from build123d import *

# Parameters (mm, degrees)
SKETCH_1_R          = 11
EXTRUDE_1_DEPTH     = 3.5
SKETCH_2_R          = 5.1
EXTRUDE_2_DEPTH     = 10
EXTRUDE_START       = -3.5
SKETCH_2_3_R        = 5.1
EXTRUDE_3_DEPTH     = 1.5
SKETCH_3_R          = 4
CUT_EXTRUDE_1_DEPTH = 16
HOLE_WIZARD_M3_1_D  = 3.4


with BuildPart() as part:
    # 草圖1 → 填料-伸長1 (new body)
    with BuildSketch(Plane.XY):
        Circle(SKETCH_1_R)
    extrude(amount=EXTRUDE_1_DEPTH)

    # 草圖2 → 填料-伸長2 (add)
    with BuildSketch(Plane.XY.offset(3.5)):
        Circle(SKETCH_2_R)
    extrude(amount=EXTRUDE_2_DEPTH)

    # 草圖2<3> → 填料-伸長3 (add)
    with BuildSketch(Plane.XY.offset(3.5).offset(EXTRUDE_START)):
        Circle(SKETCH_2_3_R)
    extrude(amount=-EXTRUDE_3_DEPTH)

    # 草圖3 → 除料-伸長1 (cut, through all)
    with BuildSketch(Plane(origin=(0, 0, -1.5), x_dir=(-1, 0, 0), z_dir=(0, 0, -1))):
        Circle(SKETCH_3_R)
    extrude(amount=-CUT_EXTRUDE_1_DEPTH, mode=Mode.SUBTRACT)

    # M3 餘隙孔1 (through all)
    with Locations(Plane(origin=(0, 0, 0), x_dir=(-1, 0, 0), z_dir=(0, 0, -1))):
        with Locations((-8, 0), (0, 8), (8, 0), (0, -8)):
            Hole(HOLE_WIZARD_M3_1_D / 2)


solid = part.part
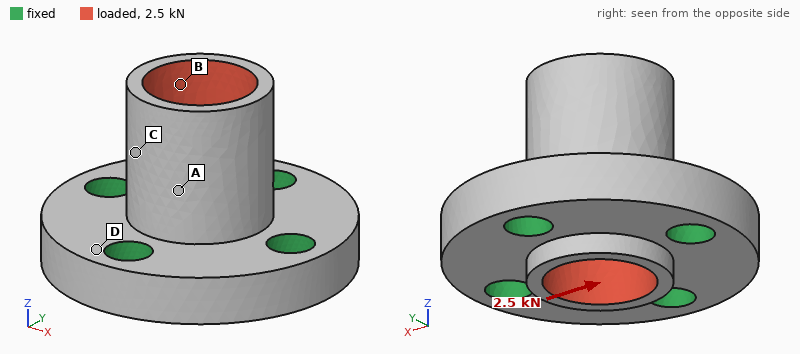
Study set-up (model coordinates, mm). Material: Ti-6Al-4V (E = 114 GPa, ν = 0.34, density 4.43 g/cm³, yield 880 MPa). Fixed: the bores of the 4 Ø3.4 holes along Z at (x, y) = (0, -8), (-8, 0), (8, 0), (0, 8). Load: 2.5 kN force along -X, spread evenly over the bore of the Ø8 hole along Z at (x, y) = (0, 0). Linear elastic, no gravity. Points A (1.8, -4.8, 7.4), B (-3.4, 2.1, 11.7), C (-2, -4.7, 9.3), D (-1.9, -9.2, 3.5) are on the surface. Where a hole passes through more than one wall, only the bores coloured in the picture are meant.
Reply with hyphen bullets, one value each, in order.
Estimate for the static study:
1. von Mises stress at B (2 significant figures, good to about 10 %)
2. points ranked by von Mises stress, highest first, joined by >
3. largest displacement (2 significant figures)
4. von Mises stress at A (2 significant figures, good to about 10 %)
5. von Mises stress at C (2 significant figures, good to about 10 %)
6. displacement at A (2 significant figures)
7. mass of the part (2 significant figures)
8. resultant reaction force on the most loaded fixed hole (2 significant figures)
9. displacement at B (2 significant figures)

- 35 MPa
- A > C > B > D
- 26 µm
- 92 MPa
- 69 MPa
- 12 µm
- 6.2 g
- 1.0 kN
- 23 µm
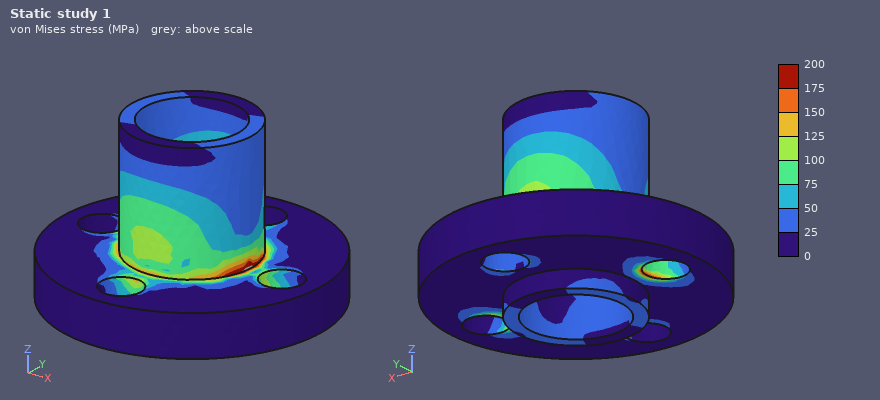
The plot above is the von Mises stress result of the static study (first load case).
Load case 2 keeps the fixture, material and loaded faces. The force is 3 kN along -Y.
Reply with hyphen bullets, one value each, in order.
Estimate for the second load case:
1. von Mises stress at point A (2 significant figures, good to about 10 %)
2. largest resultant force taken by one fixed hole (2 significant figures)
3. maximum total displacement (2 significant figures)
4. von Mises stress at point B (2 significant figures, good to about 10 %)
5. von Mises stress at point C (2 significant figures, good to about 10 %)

- 61 MPa
- 1.3 kN
- 32 µm
- 45 MPa
- 51 MPa
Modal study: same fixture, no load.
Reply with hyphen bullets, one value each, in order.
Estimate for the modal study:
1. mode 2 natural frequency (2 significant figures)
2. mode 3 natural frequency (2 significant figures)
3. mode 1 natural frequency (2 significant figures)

- 39 kHz
- 42 kHz
- 39 kHz
